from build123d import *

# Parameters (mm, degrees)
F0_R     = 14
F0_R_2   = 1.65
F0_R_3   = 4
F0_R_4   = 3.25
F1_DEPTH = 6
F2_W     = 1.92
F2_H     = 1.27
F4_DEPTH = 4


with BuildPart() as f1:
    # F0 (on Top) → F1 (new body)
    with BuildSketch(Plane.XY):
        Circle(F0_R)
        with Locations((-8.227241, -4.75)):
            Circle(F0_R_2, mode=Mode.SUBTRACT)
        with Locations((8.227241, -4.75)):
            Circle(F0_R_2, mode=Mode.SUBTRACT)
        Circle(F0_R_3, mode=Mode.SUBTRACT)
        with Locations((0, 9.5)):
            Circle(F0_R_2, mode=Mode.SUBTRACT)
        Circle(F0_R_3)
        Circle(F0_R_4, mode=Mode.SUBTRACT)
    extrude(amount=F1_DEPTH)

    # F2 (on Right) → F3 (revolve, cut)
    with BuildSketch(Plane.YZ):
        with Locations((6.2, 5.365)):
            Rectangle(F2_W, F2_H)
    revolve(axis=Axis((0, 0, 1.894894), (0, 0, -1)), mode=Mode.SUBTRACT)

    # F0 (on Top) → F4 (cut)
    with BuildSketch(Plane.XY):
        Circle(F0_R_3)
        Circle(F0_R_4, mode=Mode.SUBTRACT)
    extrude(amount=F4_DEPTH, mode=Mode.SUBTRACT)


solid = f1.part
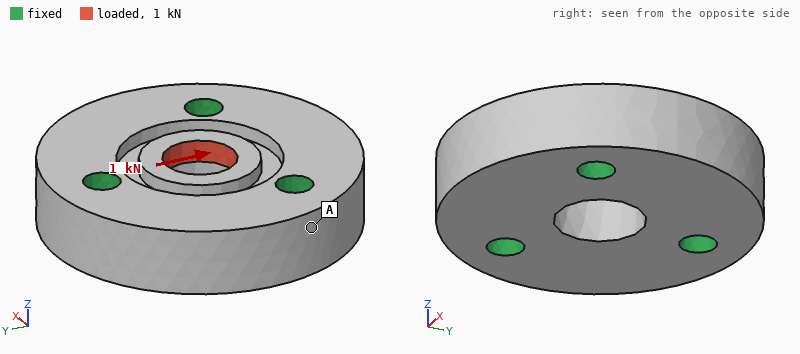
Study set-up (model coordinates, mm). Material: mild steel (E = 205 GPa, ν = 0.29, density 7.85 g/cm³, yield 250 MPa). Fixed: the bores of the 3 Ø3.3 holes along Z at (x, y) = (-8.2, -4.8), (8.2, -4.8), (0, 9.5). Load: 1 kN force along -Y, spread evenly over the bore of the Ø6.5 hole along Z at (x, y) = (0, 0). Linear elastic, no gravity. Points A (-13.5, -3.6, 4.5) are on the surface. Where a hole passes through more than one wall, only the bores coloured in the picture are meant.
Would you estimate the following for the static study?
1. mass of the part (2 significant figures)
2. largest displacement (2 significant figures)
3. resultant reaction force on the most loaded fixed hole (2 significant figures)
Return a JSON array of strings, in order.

["25 g", "1.5 µm", "340 N"]
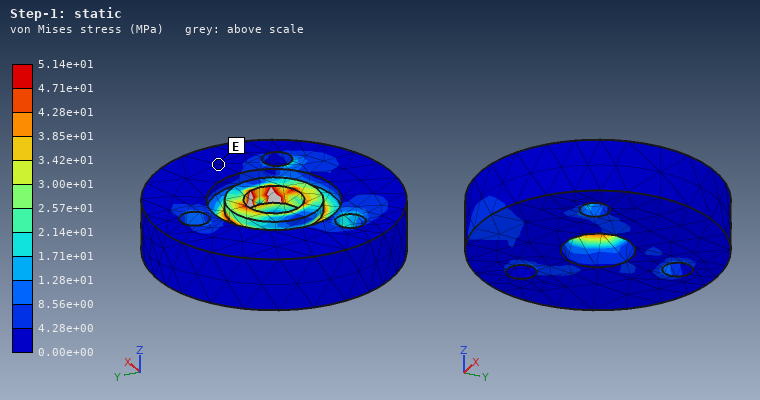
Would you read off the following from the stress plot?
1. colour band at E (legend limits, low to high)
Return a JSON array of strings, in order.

["0.00e+00 to 4.28e+00 MPa"]
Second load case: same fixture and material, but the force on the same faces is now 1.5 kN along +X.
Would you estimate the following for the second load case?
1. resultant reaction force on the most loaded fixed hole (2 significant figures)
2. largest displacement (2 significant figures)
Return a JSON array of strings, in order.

["520 N", "2.2 µm"]
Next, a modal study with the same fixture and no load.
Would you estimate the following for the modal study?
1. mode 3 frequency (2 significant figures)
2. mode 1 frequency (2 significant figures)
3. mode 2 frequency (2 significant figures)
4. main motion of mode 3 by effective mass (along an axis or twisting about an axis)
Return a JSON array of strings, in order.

["49 kHz", "46 kHz", "46 kHz", "along Z"]
